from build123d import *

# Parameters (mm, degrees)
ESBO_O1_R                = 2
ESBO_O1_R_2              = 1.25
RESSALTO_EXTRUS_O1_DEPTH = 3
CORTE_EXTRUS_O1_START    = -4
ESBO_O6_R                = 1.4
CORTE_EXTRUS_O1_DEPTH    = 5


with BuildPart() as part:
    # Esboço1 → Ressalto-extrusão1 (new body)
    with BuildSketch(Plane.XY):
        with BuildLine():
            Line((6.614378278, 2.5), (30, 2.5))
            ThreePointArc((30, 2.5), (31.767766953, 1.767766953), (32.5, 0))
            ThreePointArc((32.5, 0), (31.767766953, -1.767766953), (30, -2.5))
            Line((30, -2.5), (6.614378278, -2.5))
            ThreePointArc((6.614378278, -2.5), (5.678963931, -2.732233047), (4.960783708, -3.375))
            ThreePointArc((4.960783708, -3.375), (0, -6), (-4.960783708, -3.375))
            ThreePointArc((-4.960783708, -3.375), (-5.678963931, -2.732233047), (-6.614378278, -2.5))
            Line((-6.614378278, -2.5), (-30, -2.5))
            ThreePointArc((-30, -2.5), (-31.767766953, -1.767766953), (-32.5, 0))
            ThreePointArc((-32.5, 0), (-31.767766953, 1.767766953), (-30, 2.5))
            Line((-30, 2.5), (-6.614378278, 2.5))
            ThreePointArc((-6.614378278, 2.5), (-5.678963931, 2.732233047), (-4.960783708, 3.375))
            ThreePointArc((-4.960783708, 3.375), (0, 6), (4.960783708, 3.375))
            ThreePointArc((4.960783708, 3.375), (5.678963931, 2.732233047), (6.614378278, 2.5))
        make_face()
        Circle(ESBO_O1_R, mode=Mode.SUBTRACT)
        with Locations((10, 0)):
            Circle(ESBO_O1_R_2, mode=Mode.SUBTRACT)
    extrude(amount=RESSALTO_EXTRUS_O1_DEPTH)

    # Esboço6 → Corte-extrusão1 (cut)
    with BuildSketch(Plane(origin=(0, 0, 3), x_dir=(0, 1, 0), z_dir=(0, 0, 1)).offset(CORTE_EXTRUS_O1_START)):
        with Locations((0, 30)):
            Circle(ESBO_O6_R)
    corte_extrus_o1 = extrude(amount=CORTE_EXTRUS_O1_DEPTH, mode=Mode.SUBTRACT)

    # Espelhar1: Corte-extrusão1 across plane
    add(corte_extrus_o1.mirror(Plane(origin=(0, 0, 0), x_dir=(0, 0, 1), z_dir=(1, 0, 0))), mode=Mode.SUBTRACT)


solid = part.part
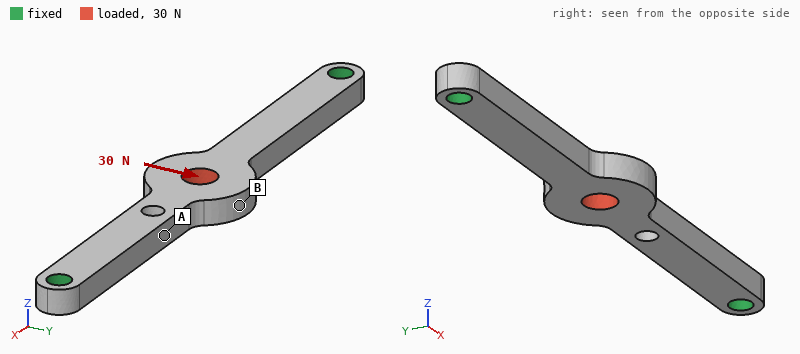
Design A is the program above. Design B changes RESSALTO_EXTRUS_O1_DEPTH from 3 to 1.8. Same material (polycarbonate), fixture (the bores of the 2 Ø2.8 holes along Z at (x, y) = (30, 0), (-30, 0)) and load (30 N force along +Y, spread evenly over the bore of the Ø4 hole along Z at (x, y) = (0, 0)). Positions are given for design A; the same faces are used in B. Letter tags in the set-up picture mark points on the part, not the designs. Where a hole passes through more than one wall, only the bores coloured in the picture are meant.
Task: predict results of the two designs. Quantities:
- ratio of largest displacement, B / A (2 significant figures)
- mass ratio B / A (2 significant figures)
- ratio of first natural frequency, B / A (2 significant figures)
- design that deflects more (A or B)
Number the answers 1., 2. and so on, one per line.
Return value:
1. 1.7
2. 0.60
3. 0.62
4. B
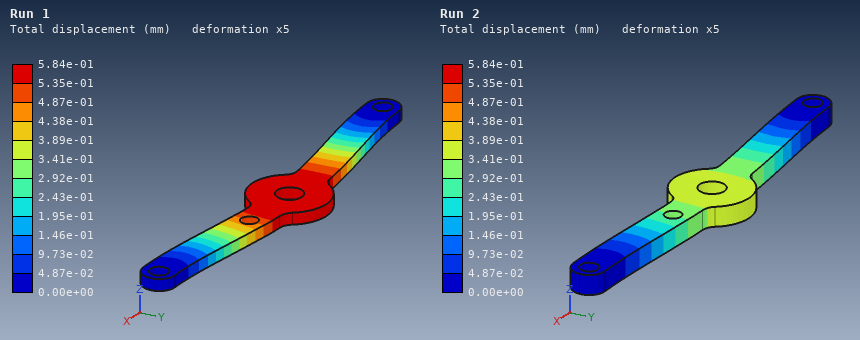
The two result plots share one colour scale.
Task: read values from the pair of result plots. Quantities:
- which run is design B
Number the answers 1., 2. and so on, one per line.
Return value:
1. Run 1
